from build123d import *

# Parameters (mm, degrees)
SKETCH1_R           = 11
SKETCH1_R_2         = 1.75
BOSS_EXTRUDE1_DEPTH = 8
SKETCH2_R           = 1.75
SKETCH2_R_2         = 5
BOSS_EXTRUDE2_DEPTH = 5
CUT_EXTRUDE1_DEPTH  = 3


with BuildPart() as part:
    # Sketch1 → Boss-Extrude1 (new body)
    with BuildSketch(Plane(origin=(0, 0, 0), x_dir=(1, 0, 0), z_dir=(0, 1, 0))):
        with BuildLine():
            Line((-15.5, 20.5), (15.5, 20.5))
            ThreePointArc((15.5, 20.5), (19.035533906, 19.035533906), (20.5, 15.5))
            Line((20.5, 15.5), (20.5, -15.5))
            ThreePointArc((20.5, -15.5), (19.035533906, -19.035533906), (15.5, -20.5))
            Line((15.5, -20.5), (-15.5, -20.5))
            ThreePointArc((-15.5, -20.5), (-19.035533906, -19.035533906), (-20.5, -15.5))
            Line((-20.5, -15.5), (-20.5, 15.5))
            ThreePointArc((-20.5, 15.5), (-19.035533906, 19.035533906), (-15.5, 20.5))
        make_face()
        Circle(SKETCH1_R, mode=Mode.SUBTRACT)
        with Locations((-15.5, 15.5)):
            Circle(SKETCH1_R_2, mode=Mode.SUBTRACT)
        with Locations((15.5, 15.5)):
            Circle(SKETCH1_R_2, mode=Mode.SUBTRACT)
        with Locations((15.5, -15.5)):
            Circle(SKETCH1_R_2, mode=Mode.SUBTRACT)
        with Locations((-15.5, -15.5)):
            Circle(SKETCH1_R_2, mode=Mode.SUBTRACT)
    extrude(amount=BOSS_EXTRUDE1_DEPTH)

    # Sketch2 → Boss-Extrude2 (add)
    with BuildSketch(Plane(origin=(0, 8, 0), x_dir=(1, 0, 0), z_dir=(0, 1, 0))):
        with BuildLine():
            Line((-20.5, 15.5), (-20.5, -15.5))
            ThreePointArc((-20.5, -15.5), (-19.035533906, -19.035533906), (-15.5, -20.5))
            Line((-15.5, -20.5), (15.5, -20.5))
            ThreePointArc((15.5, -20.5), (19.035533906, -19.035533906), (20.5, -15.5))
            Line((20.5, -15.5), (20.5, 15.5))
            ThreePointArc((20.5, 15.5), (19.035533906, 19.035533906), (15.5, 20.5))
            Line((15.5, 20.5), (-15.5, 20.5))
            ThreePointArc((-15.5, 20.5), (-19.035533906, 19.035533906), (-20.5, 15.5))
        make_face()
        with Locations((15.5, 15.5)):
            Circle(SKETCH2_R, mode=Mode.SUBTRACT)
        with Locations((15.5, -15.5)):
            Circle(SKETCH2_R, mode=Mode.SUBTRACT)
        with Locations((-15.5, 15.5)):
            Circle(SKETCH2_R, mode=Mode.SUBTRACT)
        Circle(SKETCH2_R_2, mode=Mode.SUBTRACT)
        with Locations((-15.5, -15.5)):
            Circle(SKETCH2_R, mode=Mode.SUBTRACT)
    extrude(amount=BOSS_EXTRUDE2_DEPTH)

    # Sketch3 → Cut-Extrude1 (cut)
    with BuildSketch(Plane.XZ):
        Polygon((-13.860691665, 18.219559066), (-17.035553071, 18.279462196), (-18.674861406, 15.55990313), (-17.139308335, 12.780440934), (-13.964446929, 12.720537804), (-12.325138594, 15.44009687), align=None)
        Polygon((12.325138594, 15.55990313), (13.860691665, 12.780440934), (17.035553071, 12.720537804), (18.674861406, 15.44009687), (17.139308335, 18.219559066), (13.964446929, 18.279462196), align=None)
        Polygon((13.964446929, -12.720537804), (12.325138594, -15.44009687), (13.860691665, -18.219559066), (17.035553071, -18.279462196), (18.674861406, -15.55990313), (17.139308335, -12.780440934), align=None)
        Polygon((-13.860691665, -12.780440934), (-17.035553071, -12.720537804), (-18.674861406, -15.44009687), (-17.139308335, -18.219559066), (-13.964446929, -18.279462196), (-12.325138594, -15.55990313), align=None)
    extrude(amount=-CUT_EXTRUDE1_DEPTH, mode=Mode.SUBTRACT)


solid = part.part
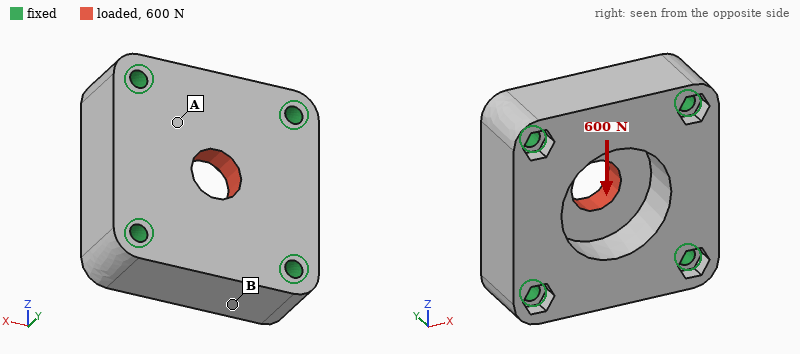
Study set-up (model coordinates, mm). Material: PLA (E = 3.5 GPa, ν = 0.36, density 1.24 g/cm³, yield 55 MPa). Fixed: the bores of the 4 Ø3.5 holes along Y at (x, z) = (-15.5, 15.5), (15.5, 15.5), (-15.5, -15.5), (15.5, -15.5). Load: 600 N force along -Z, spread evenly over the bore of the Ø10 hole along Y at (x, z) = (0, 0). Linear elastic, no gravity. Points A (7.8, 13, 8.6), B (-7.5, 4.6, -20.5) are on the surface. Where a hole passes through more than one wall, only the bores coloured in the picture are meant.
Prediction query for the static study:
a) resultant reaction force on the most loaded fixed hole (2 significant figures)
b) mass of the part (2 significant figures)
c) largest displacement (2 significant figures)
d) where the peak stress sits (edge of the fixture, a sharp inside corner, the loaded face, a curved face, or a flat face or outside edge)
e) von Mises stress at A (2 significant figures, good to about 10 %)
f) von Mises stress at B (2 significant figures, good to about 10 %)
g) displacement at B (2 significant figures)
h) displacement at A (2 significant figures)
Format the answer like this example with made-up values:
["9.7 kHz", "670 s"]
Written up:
["170 N", "22 g", "18 µm", "the loaded face", "2.7 MPa", "0.80 MPa", "5.1 µm", "8.2 µm"]
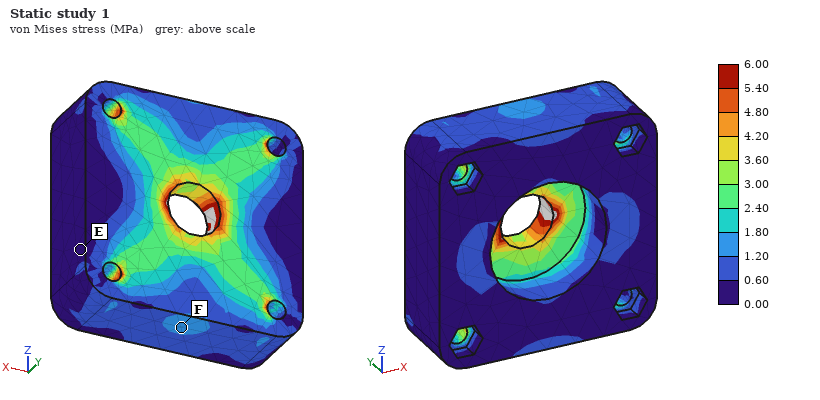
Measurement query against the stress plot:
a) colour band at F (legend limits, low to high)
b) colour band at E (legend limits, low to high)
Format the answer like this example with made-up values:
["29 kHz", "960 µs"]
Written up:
["1.20 to 1.80 MPa", "0.00 to 0.60 MPa"]
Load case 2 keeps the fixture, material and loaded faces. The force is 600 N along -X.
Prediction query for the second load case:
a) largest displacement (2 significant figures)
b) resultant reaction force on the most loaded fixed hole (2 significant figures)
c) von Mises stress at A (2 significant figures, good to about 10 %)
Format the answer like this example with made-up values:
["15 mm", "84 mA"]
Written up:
["18 µm", "170 N", "2.5 MPa"]
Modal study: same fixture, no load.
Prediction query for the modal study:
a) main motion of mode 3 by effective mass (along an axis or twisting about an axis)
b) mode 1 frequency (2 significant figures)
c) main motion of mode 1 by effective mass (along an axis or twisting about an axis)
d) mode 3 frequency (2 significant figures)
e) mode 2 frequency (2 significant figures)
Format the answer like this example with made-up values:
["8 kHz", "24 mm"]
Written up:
["twisting about X", "9600 Hz", "along Y", "12 kHz", "11 kHz"]
